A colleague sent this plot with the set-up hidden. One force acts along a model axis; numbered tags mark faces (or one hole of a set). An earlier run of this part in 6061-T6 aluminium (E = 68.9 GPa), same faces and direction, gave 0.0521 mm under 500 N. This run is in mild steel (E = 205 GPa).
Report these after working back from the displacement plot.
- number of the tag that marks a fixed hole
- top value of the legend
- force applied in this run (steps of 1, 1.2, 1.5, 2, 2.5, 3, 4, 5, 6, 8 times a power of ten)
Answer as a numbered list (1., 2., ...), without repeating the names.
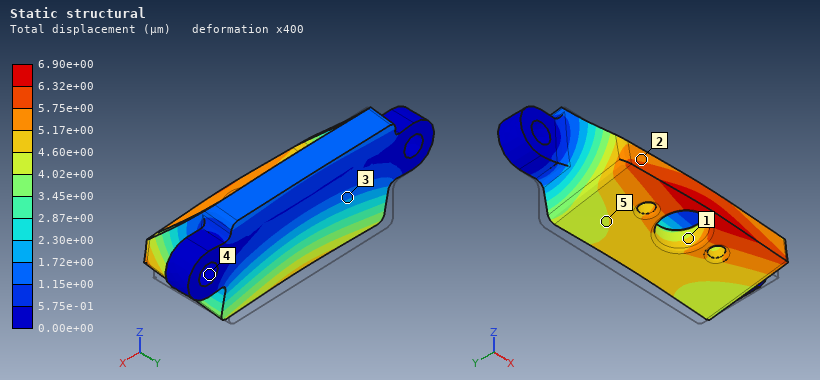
1. 4
2. 6.90e+00 µm
3. 200 N
